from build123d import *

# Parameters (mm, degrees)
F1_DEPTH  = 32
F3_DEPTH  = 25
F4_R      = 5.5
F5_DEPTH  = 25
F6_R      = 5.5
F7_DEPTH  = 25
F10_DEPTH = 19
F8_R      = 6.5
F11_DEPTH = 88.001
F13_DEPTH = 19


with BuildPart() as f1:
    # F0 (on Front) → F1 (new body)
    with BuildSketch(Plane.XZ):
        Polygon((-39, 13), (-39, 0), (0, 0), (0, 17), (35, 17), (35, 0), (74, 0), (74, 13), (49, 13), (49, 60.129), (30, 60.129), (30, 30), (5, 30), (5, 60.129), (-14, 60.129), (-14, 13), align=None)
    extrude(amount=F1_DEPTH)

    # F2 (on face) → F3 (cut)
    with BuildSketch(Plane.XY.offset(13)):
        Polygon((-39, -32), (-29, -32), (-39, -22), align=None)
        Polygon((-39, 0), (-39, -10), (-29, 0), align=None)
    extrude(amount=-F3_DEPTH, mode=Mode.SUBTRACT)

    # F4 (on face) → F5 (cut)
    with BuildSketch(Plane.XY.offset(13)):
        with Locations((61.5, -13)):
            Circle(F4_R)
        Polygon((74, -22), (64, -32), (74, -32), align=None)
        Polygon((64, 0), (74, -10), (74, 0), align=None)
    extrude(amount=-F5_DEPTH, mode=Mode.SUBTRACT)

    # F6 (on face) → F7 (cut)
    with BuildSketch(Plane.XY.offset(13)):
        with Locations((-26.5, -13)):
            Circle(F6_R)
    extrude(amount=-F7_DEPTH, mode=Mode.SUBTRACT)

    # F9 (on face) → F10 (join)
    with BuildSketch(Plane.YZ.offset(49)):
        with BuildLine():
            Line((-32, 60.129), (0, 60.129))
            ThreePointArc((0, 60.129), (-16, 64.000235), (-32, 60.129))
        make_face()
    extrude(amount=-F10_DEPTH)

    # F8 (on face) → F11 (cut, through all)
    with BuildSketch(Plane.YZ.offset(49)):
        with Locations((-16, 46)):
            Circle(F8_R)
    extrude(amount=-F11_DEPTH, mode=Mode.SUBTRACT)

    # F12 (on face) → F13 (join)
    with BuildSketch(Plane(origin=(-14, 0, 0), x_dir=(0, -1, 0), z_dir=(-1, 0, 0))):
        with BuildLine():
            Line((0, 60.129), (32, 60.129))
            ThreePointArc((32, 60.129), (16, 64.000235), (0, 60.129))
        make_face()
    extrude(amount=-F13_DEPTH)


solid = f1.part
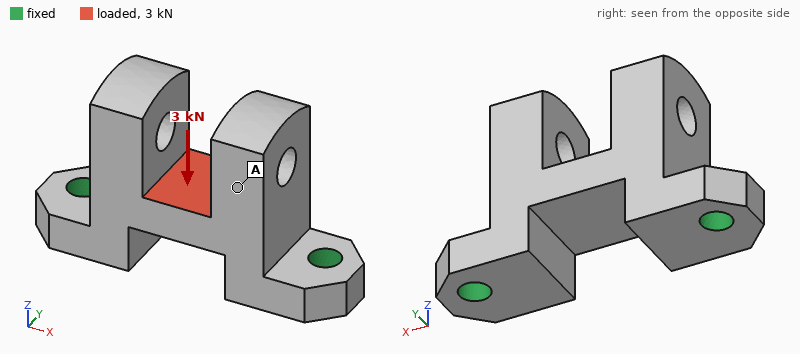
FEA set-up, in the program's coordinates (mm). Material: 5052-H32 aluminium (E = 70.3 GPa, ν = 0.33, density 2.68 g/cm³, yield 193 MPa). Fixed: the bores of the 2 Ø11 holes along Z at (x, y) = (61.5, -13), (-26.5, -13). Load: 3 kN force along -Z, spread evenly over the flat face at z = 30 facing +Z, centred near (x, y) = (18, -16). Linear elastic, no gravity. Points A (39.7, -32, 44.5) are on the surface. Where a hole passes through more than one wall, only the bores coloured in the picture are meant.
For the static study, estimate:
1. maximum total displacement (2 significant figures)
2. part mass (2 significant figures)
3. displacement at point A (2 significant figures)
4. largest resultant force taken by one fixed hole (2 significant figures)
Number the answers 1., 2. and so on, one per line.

1. 15 µm
2. 250 g
3. 10 µm
4. 2.2 kN
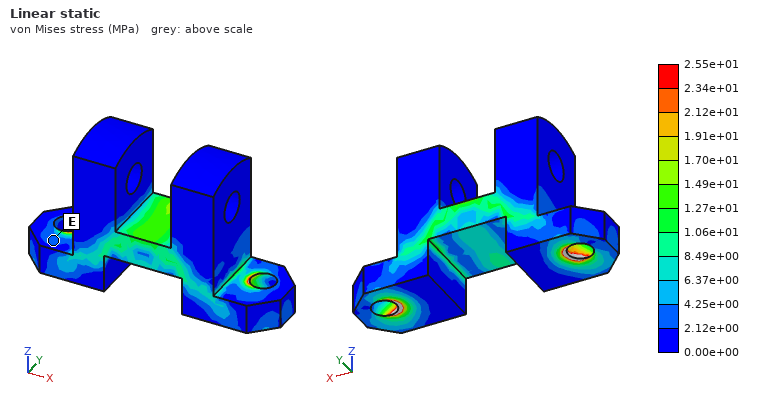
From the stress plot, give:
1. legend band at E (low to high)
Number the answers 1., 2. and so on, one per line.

1. 2.12e+00 to 4.25e+00 MPa
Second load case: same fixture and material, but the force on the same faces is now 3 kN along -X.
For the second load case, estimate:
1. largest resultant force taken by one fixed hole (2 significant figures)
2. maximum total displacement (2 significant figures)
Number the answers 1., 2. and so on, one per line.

1. 1.7 kN
2. 7.8 µm
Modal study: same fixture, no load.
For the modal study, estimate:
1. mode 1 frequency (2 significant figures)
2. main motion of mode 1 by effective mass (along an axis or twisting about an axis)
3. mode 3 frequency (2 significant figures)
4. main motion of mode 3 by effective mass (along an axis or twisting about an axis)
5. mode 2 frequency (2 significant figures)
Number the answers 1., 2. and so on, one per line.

1. 2800 Hz
2. along Y
3. 5700 Hz
4. along X
5. 4700 Hz
